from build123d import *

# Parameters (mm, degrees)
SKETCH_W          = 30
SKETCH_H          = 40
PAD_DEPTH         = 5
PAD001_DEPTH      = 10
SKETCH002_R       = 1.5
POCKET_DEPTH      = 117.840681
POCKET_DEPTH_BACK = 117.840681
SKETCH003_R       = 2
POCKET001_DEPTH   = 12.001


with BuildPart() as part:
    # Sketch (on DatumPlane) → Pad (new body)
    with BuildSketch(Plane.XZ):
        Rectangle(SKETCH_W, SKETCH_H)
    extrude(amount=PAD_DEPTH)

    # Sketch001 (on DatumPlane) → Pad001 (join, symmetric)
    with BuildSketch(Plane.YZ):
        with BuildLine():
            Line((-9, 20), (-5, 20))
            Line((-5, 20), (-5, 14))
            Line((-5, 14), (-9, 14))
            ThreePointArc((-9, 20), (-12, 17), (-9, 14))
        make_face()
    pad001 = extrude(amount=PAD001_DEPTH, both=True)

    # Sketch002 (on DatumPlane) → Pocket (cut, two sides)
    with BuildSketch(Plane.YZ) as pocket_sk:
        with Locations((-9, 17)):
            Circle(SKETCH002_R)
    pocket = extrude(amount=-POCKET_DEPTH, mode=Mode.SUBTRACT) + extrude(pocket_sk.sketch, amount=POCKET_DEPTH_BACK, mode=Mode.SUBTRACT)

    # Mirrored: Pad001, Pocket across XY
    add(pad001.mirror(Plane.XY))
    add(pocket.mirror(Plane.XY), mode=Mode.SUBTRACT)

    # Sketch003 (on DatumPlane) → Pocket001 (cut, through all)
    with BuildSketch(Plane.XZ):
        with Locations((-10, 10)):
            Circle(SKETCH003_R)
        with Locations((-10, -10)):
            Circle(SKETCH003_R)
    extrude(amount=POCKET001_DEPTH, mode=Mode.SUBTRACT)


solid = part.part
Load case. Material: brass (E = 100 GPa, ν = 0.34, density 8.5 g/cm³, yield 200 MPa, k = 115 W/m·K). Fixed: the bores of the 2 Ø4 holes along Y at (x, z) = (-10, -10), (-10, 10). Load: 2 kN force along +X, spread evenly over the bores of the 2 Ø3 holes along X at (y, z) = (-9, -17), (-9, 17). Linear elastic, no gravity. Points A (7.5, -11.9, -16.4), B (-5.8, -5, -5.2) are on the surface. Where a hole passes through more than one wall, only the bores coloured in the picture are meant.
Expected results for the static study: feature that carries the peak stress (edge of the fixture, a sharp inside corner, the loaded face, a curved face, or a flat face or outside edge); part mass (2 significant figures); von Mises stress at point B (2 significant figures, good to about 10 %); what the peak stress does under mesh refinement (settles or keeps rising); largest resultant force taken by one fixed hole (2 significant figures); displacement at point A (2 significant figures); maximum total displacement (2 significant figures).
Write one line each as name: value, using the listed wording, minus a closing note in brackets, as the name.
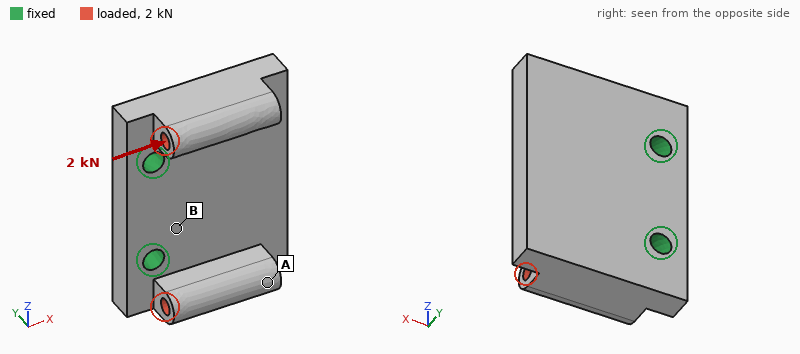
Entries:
feature that carries the peak stress: edge of the fixture
part mass: 60 g
von Mises stress at point B: 40 MPa
what the peak stress does under mesh refinement: keeps rising
largest resultant force taken by one fixed hole: 1.0 kN
displacement at point A: 38 µm
maximum total displacement: 49 µm
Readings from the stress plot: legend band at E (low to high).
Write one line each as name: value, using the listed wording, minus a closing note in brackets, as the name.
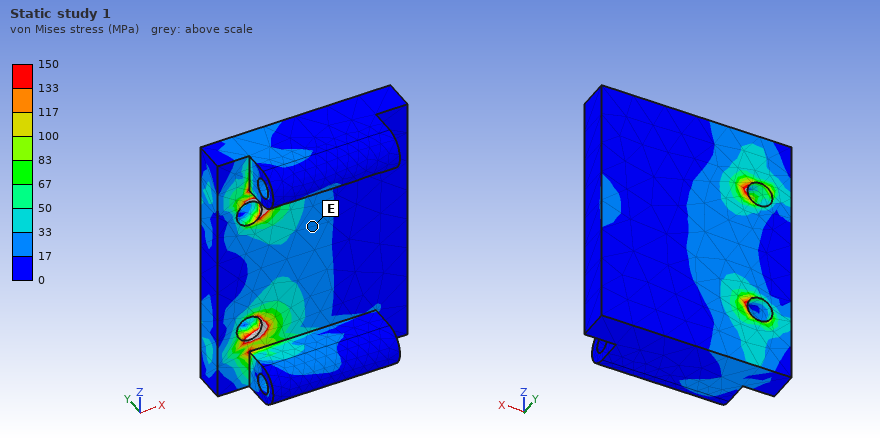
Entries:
legend band at E: 17 to 33 MPa
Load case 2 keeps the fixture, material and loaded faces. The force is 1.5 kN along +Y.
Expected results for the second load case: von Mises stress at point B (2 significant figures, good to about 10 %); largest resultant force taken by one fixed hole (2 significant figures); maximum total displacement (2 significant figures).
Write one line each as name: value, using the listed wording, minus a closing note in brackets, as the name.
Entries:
von Mises stress at point B: 38 MPa
largest resultant force taken by one fixed hole: 750 N
maximum total displacement: 53 µm
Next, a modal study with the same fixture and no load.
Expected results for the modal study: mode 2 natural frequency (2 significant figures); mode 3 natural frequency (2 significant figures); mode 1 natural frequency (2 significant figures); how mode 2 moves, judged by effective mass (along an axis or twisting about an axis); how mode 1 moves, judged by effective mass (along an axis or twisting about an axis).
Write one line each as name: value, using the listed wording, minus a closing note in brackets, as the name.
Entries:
mode 2 natural frequency: 6000 Hz
mode 3 natural frequency: 11 kHz
mode 1 natural frequency: 4400 Hz
how mode 2 moves, judged by effective mass: twisting about X
how mode 1 moves, judged by effective mass: along Y
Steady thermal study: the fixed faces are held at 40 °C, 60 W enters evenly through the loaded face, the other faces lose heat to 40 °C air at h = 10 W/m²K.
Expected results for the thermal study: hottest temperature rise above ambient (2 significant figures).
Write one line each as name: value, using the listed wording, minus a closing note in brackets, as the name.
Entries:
hottest temperature rise above ambient: 46 K
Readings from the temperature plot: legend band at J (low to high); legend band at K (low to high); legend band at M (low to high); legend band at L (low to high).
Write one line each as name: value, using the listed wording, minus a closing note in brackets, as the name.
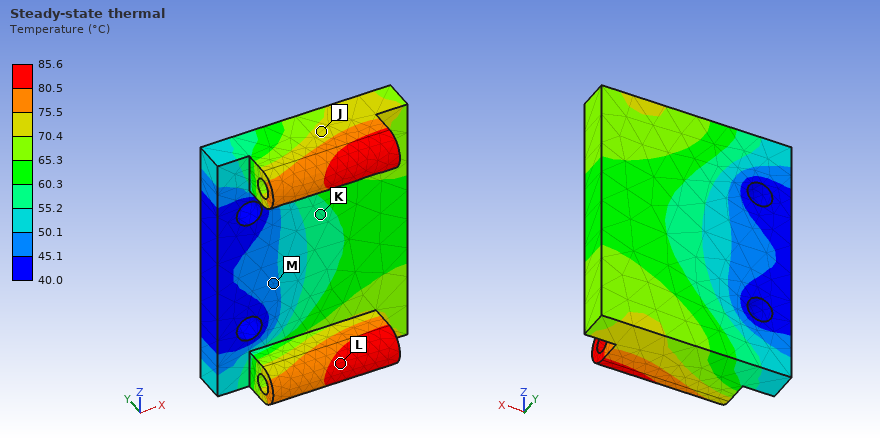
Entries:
legend band at J: 70.4 to 75.5 °C
legend band at K: 55.2 to 60.3 °C
legend band at M: 45.1 to 50.1 °C
legend band at L: 80.5 to 85.6 °C
